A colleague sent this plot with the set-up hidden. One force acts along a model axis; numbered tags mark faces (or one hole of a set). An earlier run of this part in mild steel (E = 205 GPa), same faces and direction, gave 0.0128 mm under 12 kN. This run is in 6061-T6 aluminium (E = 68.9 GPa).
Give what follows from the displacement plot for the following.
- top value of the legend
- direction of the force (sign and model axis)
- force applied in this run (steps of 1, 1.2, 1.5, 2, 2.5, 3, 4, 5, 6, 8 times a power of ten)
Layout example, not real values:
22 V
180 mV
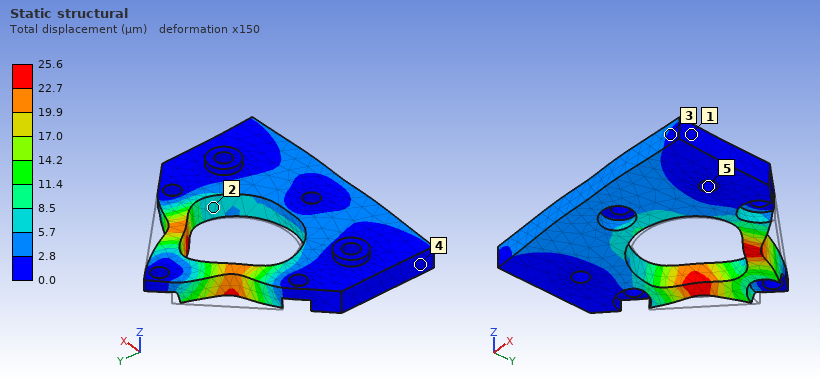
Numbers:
25.6 µm
-Y
8 kN
